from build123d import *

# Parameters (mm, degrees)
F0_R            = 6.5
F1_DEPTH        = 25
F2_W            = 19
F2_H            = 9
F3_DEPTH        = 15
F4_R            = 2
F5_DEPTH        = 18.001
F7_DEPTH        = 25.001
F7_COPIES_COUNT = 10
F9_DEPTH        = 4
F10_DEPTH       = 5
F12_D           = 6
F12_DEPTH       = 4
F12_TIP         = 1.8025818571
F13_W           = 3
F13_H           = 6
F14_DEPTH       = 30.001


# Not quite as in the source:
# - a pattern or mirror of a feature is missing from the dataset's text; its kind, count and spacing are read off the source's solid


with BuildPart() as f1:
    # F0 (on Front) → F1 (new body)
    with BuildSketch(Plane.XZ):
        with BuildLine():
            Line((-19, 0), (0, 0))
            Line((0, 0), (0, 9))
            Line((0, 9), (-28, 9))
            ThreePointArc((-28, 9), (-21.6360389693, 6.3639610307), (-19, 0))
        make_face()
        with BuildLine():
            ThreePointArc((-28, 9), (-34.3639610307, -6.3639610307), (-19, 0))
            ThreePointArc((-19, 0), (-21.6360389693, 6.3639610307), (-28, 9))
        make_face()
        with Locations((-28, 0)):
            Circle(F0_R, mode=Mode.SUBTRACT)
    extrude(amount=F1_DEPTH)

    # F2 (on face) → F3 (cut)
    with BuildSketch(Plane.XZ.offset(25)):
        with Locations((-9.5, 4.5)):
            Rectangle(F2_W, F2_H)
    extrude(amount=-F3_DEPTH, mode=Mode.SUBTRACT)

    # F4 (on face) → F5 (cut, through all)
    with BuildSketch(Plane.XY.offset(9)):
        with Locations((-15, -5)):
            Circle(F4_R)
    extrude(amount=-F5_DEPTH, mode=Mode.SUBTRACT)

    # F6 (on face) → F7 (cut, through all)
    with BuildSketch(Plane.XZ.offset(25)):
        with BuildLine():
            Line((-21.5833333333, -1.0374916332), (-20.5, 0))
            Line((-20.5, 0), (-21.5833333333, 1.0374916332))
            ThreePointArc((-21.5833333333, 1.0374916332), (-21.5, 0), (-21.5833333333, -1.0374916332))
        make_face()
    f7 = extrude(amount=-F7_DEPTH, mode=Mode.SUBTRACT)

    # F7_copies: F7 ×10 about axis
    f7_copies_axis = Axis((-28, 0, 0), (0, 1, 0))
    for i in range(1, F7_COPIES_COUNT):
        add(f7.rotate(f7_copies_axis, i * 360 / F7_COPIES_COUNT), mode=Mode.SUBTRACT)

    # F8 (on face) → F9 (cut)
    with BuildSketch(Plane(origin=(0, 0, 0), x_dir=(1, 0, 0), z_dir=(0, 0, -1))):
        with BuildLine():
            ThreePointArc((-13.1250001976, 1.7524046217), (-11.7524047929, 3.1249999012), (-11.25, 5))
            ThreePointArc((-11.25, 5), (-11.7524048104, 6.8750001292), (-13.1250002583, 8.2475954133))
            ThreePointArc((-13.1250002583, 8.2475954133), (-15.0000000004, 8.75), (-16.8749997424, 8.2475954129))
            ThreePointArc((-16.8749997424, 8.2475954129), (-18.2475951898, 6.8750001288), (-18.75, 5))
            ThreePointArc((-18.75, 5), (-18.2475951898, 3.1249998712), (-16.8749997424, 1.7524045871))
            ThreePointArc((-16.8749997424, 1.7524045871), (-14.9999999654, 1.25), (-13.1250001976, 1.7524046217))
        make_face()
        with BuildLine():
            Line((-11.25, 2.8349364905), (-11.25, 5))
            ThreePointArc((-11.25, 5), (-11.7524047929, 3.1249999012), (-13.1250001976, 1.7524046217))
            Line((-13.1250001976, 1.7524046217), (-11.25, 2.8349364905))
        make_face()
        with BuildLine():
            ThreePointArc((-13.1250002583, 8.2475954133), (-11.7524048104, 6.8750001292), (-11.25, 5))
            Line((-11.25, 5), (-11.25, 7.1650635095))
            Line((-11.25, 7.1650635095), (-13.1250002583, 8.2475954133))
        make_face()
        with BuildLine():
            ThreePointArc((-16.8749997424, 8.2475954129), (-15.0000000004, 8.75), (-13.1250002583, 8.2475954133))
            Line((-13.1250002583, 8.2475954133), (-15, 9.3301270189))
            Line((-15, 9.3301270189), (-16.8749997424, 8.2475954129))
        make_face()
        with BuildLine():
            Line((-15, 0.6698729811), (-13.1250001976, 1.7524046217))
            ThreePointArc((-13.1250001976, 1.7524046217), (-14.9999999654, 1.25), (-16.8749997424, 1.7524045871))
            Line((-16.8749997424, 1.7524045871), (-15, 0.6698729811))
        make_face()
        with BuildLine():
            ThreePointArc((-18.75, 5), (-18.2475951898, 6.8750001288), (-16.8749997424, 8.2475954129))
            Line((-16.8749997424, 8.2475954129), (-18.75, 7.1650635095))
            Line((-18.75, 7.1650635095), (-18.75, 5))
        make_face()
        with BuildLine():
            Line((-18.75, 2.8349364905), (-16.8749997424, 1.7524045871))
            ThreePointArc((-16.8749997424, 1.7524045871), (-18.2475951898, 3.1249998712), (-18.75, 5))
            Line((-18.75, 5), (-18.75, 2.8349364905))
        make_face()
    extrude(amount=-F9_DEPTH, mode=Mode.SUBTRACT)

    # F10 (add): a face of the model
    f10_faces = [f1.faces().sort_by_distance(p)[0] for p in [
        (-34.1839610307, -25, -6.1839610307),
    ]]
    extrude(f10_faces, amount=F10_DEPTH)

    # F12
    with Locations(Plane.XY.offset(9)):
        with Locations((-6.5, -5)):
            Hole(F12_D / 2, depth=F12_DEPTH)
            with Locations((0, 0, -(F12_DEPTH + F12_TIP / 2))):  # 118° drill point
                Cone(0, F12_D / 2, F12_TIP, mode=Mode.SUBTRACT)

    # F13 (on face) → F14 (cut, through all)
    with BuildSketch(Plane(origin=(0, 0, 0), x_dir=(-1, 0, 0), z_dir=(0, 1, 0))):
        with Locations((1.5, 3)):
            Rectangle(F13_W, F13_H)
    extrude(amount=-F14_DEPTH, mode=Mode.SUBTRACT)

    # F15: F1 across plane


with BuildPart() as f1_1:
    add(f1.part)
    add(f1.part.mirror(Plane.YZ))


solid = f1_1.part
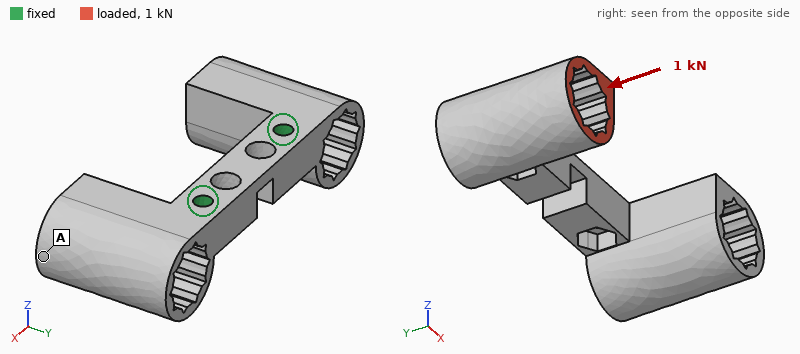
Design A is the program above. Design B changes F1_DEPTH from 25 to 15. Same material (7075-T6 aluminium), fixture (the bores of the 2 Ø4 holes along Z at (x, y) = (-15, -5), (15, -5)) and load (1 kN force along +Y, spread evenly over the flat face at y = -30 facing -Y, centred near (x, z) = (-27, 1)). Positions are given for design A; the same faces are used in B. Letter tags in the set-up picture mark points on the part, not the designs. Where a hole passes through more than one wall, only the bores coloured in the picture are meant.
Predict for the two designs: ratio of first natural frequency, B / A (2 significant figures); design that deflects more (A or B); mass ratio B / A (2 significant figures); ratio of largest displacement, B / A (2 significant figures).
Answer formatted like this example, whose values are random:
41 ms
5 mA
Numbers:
1.3
A
0.74
0.85
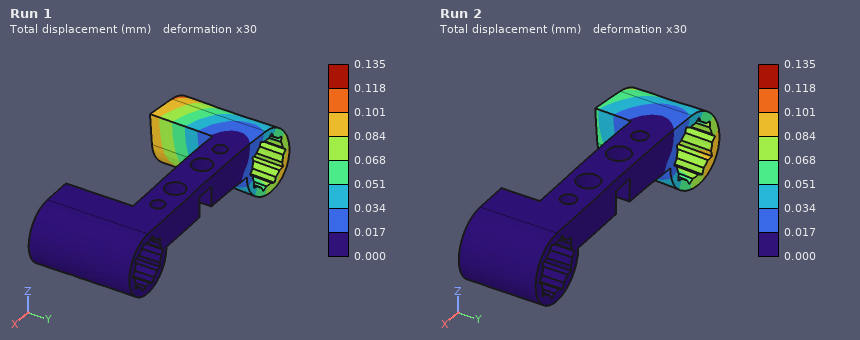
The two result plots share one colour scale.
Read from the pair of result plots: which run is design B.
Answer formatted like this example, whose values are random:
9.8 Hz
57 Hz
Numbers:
Run 2
